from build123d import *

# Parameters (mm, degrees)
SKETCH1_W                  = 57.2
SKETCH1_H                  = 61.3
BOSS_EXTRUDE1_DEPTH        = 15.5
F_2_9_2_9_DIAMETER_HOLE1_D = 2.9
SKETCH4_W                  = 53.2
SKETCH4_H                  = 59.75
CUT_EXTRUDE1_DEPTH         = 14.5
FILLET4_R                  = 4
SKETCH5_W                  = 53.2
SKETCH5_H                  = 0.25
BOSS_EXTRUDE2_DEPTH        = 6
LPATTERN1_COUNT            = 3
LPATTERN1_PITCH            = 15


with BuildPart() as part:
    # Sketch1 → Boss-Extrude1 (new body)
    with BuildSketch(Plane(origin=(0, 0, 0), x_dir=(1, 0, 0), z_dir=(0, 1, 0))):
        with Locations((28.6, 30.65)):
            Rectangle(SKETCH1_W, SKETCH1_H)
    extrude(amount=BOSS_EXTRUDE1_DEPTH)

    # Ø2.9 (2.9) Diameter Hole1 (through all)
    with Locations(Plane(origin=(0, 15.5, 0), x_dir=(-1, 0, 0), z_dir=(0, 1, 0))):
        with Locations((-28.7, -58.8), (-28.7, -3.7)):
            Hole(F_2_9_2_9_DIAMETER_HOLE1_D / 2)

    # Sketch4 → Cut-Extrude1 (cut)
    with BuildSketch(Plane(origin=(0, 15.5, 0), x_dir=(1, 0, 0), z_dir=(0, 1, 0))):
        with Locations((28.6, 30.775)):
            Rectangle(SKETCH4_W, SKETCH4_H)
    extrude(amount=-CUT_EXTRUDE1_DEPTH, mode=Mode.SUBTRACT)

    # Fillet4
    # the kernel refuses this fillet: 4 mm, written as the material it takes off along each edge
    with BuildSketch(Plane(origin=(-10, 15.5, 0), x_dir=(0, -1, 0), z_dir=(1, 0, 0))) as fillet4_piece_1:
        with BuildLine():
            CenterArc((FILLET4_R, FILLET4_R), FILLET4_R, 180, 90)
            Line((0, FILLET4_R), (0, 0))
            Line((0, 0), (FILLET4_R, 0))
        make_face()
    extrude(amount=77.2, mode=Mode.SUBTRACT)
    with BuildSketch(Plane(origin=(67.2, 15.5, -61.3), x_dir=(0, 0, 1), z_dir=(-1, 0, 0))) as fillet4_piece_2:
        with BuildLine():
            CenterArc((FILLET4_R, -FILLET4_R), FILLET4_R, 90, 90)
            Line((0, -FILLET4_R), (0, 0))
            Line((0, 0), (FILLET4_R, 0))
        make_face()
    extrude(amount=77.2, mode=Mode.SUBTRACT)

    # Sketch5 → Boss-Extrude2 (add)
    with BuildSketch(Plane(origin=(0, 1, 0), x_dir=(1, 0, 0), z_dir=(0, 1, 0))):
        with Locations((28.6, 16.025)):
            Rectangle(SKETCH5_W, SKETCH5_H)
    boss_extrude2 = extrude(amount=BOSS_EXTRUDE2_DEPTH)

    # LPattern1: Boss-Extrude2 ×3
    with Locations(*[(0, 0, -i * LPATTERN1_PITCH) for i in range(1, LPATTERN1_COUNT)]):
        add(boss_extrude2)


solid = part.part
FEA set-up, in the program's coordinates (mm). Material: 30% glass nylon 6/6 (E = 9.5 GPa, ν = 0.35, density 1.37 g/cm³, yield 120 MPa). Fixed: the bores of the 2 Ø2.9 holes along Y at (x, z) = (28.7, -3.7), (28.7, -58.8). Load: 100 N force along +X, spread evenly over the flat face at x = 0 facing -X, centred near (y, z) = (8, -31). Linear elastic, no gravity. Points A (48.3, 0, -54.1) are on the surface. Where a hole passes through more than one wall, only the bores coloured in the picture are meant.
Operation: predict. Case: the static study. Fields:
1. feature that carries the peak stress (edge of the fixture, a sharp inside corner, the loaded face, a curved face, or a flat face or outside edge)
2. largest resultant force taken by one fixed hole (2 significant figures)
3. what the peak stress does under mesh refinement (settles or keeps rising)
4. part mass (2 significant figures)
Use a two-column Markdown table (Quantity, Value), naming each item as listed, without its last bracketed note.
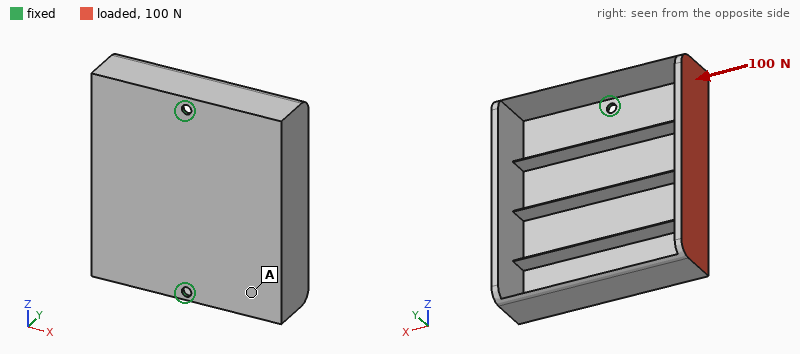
| Quantity | Value |
|---|---|
| feature that carries the peak stress | edge of the fixture |
| largest resultant force taken by one fixed hole | 51 N |
| what the peak stress does under mesh refinement | keeps rising |
| part mass | 11 g |
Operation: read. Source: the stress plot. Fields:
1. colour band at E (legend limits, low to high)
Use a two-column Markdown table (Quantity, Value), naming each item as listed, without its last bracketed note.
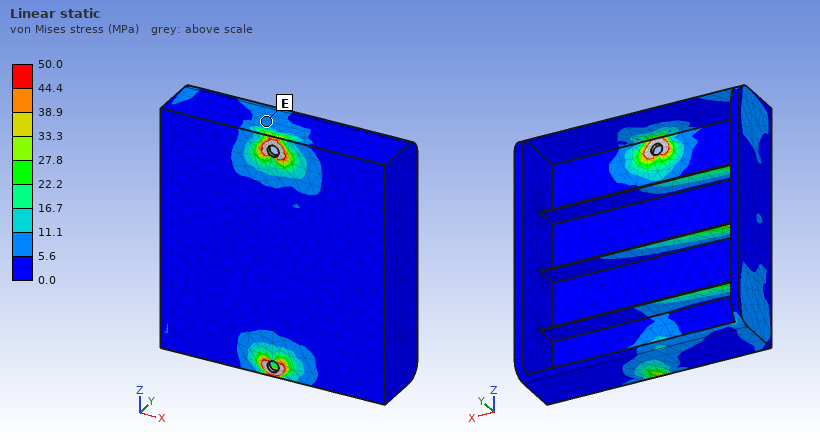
| Quantity | Value |
|---|---|
| colour band at E | 5.6 to 11.1 MPa |
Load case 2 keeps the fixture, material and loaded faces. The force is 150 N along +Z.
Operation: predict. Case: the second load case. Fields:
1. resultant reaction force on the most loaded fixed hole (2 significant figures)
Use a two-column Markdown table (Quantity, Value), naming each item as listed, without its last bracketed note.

| Quantity | Value |
|---|---|
| resultant reaction force on the most loaded fixed hole | 110 N |
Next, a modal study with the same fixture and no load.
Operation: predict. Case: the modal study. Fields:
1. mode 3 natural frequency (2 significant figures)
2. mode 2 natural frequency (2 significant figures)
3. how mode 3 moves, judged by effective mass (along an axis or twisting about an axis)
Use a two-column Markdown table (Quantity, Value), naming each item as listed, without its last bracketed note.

| Quantity | Value |
|---|---|
| mode 3 natural frequency | 1500 Hz |
| mode 2 natural frequency | 700 Hz |
| how mode 3 moves, judged by effective mass | along Y |
